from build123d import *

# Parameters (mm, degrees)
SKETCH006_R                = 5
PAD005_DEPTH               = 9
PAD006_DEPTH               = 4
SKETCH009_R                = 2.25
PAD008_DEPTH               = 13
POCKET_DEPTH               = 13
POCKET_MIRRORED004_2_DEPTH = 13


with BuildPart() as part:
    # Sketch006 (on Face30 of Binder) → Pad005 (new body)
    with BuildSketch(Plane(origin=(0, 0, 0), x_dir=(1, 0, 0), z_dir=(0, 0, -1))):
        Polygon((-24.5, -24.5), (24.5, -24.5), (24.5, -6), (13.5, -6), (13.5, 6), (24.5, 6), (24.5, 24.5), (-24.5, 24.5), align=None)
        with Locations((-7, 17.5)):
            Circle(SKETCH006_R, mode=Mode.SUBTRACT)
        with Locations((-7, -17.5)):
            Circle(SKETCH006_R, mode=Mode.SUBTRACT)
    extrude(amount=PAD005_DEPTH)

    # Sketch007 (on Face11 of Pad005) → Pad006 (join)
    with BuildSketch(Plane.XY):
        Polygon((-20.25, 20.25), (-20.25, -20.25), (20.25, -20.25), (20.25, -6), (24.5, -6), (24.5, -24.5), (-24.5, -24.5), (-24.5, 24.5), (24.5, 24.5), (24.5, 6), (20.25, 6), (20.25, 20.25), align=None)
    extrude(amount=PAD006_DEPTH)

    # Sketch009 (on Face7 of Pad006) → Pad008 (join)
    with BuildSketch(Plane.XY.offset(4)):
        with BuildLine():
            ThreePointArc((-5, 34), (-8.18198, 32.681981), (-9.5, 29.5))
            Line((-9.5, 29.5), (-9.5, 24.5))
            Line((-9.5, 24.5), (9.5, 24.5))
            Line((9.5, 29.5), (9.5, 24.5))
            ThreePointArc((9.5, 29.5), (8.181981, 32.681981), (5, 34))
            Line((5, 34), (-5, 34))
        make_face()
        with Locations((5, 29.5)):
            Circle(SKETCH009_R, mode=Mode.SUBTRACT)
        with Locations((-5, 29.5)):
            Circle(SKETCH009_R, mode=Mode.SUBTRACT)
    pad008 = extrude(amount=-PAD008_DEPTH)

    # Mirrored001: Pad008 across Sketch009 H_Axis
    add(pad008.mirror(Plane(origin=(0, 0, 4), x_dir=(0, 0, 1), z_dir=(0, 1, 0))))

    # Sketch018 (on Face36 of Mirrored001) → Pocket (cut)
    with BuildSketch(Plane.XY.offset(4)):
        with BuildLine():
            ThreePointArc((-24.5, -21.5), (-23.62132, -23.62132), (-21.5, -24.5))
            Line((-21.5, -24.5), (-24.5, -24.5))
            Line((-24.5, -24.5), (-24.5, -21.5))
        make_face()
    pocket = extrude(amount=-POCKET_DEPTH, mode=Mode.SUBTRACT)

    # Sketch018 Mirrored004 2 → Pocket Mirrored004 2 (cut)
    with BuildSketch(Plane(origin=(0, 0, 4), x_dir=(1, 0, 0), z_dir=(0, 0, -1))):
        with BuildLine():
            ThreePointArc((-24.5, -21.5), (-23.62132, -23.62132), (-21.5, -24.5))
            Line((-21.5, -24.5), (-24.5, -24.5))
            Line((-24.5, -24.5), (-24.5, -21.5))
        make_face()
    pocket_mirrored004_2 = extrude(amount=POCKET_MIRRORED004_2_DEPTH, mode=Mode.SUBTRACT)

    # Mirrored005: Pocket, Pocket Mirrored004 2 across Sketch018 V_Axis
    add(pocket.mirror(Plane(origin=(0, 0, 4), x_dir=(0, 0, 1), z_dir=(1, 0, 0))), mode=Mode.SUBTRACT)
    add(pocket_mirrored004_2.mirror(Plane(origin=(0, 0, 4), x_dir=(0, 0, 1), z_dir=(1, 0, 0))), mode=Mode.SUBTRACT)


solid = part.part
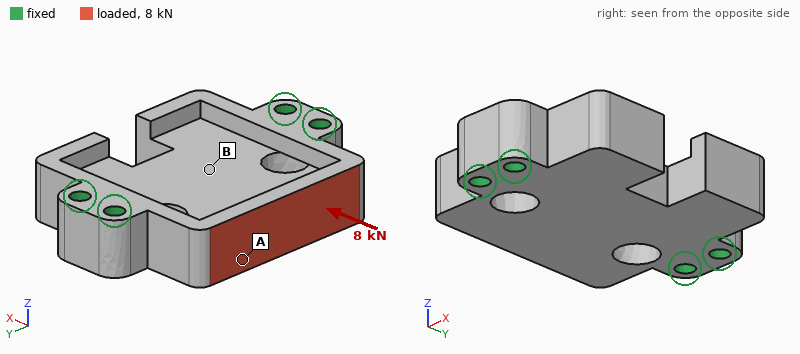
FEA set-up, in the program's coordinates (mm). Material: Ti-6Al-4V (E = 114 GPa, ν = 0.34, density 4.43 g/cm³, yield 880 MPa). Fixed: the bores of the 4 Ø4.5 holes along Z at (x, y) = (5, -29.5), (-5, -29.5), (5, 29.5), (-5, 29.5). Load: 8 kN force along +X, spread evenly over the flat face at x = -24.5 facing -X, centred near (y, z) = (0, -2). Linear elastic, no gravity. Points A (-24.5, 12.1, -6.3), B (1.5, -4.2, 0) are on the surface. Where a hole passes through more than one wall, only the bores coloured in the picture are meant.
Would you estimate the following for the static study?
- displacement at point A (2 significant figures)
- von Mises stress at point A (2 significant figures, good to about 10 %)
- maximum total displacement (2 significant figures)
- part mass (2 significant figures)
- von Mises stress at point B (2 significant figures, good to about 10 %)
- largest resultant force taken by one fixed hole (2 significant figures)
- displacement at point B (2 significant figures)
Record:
12 µm
32 MPa
24 µm
110 g
12 MPa
2.7 kN
11 µm
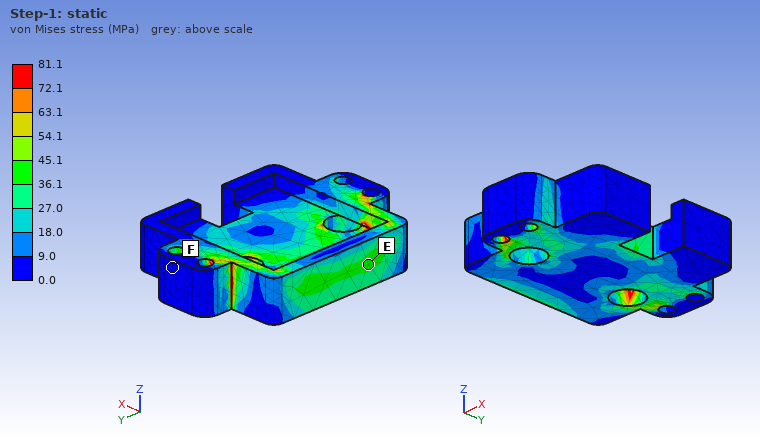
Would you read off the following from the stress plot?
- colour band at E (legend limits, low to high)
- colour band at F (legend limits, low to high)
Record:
36.1 to 45.1 MPa
0.0 to 9.0 MPa
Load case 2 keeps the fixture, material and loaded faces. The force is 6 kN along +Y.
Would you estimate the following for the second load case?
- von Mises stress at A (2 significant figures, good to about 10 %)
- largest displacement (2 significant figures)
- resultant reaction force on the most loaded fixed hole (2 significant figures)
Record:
20 MPa
18 µm
2.3 kN
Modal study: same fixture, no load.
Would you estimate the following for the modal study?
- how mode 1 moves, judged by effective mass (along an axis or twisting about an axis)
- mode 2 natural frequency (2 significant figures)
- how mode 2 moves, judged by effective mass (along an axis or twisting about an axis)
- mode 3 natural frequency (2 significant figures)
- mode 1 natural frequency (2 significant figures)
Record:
along Z
10 kHz
along Z
14 kHz
8300 Hz
